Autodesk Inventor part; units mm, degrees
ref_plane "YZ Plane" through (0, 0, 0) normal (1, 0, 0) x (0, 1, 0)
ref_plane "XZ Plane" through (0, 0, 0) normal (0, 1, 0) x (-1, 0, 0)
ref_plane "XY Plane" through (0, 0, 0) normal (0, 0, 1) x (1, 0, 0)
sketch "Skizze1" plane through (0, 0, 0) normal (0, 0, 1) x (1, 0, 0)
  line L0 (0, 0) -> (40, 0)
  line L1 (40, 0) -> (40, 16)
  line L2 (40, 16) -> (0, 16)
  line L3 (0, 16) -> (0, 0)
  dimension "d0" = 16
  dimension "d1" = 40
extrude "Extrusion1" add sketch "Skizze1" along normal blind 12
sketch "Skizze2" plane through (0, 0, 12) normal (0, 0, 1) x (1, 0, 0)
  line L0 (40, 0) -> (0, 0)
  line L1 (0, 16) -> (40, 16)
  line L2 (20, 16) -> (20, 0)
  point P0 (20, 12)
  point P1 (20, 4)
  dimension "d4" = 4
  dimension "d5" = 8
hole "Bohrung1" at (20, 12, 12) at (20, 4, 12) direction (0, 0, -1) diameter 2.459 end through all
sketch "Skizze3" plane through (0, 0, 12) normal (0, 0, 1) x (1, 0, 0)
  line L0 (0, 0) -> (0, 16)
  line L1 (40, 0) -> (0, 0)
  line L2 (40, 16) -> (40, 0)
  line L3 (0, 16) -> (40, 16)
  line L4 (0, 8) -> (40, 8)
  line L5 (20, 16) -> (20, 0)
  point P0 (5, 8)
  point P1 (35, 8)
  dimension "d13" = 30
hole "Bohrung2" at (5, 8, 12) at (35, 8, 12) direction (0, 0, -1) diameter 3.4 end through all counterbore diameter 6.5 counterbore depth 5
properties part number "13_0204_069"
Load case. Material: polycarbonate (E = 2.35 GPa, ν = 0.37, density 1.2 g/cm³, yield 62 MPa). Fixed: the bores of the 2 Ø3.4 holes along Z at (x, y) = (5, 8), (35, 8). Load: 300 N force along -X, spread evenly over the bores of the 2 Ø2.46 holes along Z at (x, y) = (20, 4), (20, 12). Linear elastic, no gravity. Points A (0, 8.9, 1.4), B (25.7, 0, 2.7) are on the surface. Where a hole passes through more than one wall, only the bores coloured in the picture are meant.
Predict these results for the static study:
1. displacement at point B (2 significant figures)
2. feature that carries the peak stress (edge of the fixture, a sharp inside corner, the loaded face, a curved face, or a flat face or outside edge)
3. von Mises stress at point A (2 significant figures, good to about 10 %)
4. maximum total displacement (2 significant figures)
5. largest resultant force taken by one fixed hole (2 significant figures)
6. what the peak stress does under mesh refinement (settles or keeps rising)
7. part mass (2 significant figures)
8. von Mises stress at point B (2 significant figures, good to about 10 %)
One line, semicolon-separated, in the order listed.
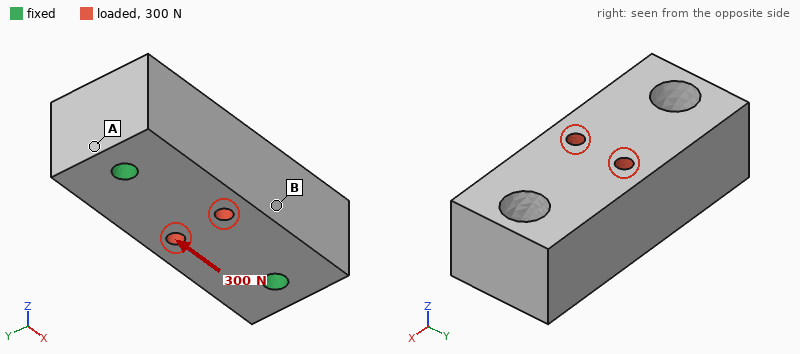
6.3 µm; edge of the fixture; 1.2 MPa; 9.5 µm; 150 N; keeps rising; 8.5 g; 0.60 MPa
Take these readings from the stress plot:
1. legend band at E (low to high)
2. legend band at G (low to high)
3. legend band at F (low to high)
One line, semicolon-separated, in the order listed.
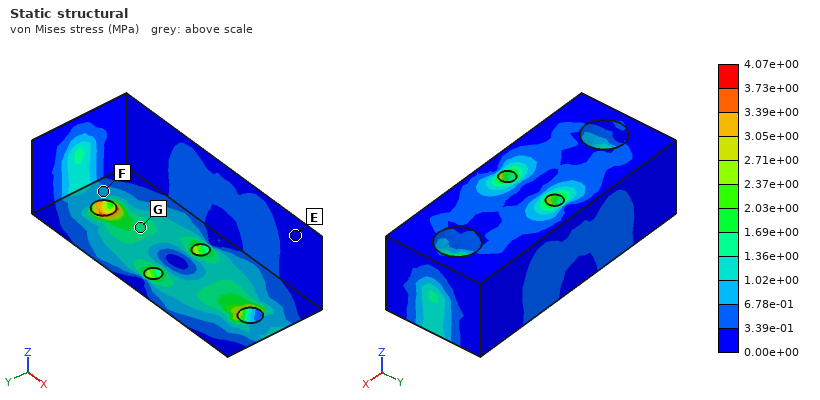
0.00e+00 to 3.39e-01 MPa; 1.36e+00 to 1.69e+00 MPa; 6.78e-01 to 1.02e+00 MPa
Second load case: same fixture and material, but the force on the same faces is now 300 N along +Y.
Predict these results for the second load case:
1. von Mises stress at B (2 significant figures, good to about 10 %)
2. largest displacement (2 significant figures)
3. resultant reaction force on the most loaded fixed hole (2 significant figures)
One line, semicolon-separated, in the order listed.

2.3 MPa; 43 µm; 150 N
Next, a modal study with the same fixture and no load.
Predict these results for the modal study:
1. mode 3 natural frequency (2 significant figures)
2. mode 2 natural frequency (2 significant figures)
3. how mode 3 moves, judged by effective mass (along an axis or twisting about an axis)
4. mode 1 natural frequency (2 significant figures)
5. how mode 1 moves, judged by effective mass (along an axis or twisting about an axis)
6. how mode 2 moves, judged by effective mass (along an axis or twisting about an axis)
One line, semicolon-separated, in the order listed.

9300 Hz; 8100 Hz; along Y; 6500 Hz; along Y; along Z
